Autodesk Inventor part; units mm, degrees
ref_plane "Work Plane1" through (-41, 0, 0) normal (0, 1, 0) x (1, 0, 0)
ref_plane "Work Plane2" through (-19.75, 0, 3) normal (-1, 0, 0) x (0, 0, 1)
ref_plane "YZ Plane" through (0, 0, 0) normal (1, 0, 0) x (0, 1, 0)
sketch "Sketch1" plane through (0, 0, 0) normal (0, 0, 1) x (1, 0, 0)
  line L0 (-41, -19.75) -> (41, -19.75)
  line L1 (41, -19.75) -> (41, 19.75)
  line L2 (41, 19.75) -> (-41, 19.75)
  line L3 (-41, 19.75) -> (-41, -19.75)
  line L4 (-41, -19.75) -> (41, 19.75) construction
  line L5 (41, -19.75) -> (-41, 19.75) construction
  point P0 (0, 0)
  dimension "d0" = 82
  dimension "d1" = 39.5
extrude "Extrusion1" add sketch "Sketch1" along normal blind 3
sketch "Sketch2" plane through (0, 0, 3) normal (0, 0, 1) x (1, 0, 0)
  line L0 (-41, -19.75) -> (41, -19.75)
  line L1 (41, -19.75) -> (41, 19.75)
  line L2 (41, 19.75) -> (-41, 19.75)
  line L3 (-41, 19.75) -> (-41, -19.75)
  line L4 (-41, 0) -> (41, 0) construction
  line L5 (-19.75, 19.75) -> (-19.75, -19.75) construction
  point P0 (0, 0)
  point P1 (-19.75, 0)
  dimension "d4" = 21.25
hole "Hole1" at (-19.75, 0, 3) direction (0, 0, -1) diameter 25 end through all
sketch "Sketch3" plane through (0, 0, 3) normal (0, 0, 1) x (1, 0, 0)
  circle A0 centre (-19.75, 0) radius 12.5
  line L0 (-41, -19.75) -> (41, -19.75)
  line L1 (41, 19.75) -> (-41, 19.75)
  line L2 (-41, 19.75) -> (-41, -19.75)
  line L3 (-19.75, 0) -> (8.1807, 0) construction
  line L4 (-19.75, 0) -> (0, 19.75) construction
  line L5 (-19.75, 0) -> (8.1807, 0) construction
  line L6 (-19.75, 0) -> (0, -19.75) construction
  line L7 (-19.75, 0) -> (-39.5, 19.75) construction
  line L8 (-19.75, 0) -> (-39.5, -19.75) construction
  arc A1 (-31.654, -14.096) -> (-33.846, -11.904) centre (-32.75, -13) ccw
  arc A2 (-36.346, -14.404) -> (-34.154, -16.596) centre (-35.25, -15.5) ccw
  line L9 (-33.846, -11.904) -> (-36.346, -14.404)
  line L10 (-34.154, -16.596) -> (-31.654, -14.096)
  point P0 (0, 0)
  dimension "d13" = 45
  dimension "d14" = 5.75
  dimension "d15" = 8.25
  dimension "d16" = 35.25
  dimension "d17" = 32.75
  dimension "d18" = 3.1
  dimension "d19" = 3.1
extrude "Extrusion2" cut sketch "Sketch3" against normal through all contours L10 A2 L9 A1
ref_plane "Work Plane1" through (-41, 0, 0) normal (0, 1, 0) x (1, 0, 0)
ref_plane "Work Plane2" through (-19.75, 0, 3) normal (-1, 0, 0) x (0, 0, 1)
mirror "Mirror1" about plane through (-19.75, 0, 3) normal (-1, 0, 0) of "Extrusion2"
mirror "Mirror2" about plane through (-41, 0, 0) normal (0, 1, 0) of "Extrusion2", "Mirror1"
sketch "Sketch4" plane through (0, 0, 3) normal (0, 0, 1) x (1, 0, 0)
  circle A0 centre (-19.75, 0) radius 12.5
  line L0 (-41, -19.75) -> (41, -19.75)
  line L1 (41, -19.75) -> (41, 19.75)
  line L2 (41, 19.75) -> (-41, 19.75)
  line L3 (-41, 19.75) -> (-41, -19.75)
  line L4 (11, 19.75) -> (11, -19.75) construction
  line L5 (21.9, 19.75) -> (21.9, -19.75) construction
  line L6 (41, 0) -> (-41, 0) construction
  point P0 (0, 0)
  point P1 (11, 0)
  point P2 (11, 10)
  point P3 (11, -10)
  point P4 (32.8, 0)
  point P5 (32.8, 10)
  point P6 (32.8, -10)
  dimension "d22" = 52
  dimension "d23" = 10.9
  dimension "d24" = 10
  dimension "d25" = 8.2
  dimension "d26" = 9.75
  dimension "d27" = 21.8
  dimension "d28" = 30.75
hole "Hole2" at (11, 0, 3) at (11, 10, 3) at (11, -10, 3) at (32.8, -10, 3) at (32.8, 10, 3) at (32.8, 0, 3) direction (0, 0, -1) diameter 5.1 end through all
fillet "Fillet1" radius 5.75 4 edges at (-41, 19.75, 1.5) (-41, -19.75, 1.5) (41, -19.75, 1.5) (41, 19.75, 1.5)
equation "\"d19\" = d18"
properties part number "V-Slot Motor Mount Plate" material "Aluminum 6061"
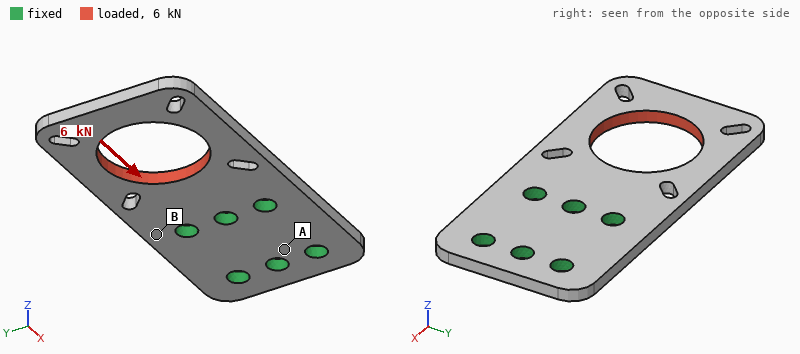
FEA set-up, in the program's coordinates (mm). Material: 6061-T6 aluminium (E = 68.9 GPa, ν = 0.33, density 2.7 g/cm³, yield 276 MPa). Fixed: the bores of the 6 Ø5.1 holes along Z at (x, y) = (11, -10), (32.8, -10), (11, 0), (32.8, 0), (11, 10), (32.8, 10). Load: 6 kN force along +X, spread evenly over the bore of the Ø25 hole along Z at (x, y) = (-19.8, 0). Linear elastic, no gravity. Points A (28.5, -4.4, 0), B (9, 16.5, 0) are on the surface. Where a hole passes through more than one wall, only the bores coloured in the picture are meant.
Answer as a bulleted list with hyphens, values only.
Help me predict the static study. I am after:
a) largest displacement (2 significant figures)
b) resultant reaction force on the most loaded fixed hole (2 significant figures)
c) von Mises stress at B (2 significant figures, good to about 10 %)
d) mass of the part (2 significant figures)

- 95 µm
- 2.2 kN
- 50 MPa
- 20 g
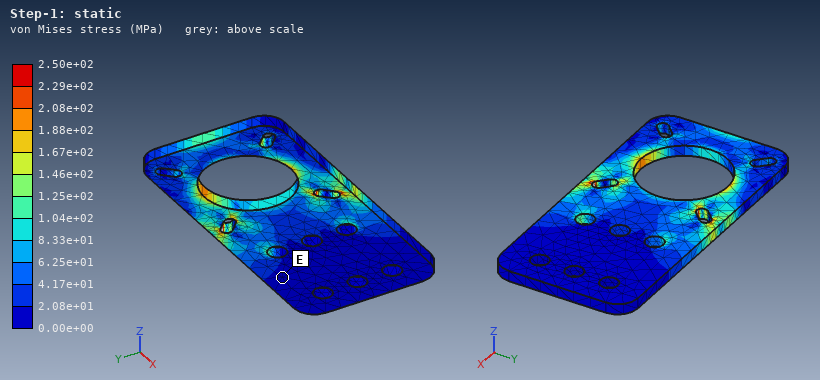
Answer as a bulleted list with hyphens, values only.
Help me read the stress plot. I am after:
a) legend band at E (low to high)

- 0.00e+00 to 2.08e+01 MPa
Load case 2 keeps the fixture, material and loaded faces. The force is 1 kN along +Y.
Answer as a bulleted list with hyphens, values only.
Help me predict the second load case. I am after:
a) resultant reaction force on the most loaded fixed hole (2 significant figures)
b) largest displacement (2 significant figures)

- 990 N
- 85 µm
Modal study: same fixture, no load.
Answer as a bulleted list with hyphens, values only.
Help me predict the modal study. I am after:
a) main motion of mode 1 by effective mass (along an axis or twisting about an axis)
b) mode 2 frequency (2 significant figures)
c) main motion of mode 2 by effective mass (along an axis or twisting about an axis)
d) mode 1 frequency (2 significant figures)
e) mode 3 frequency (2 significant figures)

- along Z
- 2300 Hz
- twisting about X
- 950 Hz
- 5500 Hz
